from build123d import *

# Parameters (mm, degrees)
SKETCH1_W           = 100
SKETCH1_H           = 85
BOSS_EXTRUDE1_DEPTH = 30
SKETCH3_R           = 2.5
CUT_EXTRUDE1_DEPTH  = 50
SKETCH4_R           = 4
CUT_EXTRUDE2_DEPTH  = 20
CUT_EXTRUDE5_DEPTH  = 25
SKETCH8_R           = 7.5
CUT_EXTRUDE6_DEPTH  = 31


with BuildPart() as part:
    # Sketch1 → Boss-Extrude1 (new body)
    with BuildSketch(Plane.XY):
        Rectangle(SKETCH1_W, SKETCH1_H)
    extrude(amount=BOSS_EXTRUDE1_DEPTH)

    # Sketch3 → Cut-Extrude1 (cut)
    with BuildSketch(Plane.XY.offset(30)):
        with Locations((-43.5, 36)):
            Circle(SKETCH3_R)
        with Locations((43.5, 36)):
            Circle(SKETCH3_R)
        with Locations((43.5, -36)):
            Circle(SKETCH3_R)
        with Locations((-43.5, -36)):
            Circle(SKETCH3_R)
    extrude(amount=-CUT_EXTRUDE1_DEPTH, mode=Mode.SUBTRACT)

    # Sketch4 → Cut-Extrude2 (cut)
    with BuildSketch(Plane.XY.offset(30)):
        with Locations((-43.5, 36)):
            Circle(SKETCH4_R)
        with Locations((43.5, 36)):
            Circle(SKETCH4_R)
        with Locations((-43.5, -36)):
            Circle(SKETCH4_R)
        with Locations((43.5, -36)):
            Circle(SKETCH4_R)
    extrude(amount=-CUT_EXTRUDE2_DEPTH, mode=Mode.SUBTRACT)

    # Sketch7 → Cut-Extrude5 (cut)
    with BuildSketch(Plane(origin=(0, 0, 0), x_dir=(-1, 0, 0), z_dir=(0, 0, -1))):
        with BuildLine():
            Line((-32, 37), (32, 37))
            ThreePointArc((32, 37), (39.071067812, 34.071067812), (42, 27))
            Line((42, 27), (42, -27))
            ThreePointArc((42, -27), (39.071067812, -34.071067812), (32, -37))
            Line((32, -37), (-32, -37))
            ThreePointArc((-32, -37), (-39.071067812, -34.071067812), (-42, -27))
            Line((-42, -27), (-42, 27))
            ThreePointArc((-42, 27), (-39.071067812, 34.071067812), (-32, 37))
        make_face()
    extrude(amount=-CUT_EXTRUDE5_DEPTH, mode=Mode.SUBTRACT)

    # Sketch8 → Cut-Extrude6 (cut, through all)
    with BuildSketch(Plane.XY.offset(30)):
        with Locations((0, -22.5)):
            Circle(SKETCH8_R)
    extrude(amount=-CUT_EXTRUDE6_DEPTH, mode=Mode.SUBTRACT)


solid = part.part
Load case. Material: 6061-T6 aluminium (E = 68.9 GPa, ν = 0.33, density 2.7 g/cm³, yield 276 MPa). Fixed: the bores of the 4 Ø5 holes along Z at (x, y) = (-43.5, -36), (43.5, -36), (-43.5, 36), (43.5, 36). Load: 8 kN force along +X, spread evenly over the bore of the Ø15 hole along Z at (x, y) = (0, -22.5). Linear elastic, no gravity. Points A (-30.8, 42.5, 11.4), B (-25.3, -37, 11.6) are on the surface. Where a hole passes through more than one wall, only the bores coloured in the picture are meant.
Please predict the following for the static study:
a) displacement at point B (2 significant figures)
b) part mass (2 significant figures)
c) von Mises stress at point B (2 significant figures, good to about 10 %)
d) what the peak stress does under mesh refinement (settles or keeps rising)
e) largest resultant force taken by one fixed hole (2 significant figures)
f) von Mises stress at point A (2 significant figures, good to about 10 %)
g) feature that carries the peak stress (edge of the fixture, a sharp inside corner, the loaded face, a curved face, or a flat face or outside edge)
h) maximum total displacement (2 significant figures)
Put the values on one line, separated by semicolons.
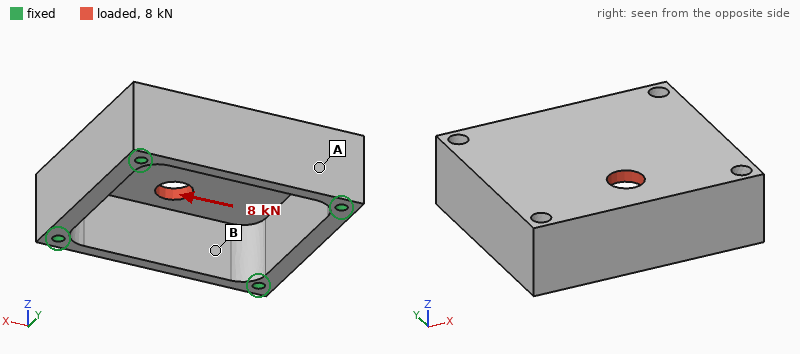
9.1 µm; 260 g; 22 MPa; keeps rising; 2.9 kN; 8.2 MPa; edge of the fixture; 27 µm
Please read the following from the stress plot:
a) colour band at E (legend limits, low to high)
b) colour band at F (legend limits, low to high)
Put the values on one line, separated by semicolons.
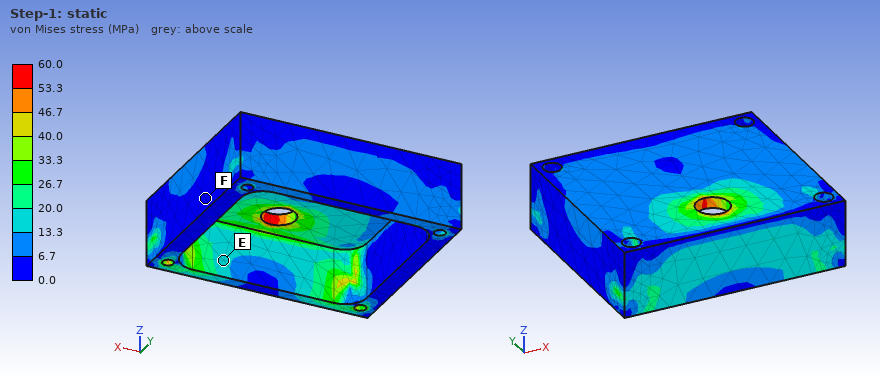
13.3 to 20.0 MPa; 0.0 to 6.7 MPa
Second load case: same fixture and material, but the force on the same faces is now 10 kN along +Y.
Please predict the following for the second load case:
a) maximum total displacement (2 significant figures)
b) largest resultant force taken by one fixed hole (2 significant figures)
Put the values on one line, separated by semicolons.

56 µm; 2.9 kN
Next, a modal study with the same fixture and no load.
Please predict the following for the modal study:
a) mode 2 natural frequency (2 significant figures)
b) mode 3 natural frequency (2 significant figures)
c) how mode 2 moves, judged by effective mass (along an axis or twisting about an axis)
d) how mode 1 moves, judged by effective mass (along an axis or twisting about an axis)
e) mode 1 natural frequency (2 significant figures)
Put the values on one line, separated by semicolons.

6700 Hz; 7500 Hz; along Y; along Z; 4700 Hz
